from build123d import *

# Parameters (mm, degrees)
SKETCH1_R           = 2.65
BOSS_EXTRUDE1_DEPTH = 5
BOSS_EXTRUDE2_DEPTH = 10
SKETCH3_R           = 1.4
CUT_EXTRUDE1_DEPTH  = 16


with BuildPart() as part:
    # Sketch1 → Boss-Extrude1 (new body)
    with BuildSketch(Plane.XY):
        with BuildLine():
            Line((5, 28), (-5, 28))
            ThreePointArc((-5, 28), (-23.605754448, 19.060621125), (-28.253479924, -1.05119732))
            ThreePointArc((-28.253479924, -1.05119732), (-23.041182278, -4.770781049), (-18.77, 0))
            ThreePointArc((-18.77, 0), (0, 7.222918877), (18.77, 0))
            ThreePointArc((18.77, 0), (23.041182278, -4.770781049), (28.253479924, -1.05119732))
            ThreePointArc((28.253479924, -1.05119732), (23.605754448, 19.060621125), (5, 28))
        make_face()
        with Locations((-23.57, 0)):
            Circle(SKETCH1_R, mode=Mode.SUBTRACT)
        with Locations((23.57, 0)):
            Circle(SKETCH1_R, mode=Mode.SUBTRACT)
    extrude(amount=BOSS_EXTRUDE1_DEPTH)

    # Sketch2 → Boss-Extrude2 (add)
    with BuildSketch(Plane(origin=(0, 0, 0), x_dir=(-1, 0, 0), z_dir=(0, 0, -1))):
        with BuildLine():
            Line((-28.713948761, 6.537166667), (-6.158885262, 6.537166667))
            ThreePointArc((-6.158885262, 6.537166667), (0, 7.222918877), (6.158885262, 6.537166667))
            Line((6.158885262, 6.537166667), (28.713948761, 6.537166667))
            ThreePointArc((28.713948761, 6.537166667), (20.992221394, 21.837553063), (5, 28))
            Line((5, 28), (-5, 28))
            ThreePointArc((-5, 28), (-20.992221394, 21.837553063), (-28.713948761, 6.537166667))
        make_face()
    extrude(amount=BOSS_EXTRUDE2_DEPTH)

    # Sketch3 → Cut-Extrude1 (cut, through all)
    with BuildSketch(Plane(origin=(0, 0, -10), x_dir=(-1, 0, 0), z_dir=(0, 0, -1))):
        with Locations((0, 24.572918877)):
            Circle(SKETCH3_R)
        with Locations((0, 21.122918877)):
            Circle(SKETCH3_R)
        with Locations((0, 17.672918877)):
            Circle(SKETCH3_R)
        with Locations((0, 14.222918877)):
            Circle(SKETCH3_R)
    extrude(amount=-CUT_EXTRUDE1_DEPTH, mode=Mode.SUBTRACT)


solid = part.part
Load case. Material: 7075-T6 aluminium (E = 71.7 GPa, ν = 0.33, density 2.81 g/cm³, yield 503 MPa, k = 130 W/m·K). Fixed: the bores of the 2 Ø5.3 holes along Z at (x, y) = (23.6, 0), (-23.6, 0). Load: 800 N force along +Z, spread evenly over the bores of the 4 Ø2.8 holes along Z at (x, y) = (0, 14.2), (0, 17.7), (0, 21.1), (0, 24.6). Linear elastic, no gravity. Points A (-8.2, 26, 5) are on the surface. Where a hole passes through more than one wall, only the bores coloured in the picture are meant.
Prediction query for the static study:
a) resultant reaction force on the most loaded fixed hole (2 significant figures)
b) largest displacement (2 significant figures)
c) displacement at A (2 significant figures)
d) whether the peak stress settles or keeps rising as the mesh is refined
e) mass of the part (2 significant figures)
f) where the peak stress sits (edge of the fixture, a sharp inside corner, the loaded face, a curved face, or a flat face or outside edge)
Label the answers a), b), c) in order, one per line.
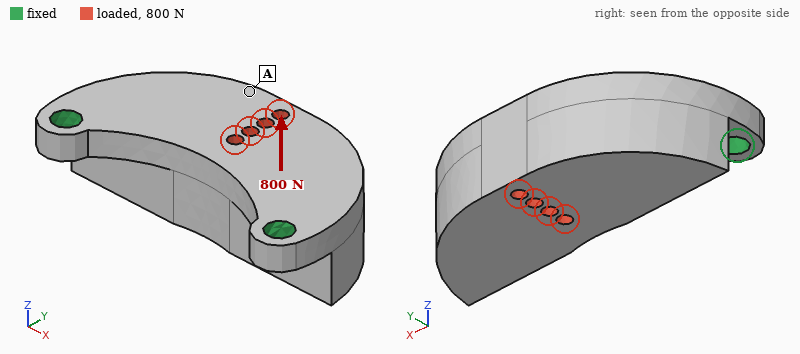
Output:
a) 430 N
b) 0.13 mm
c) 0.10 mm
d) keeps rising
e) 44 g
f) edge of the fixture
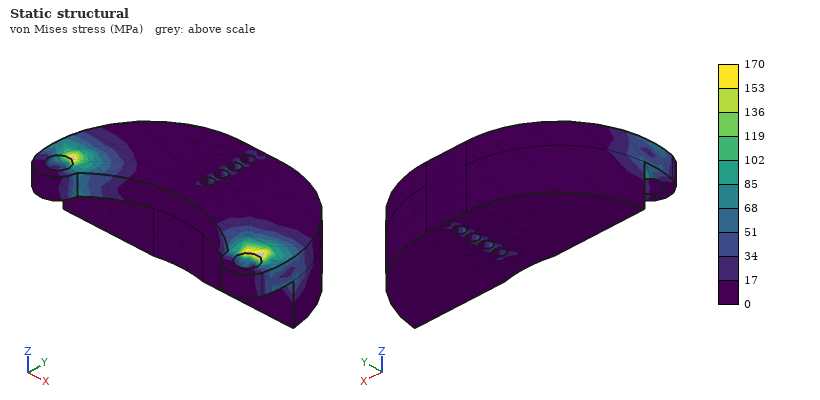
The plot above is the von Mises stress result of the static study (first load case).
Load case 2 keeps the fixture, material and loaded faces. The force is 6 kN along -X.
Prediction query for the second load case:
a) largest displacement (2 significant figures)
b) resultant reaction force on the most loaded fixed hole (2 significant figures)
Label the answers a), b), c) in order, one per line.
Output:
a) 25 µm
b) 3.7 kN
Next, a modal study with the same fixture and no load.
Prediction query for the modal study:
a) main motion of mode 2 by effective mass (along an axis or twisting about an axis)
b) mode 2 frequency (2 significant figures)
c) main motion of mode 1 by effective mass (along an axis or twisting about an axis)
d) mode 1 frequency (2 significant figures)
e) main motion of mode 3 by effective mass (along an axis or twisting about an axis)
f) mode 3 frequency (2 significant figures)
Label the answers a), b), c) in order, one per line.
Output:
a) along X
b) 13 kHz
c) along Z
d) 2800 Hz
e) along X
f) 14 kHz
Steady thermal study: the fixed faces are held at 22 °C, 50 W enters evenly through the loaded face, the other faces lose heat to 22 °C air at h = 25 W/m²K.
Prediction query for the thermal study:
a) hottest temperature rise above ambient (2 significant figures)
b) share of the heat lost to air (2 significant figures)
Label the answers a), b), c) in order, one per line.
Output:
a) 40 K
b) 5.9 %
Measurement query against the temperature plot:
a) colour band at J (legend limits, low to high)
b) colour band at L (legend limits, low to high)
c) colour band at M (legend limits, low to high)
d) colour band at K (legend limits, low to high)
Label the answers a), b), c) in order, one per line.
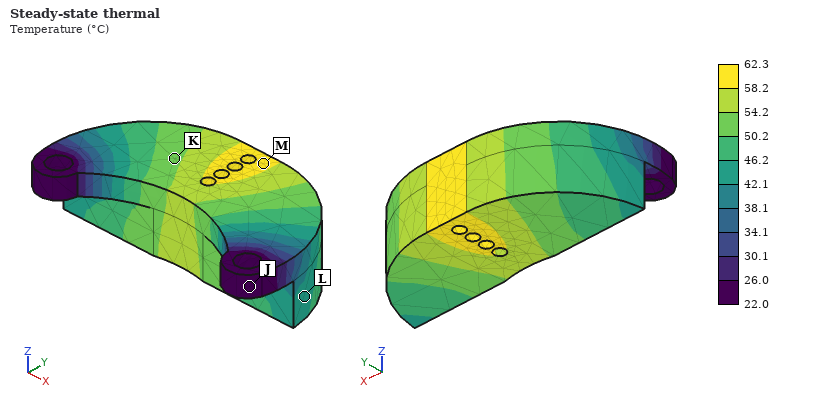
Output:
a) 22.0 to 26.0 °C
b) 42.1 to 46.2 °C
c) 58.2 to 62.3 °C
d) 50.2 to 54.2 °C
